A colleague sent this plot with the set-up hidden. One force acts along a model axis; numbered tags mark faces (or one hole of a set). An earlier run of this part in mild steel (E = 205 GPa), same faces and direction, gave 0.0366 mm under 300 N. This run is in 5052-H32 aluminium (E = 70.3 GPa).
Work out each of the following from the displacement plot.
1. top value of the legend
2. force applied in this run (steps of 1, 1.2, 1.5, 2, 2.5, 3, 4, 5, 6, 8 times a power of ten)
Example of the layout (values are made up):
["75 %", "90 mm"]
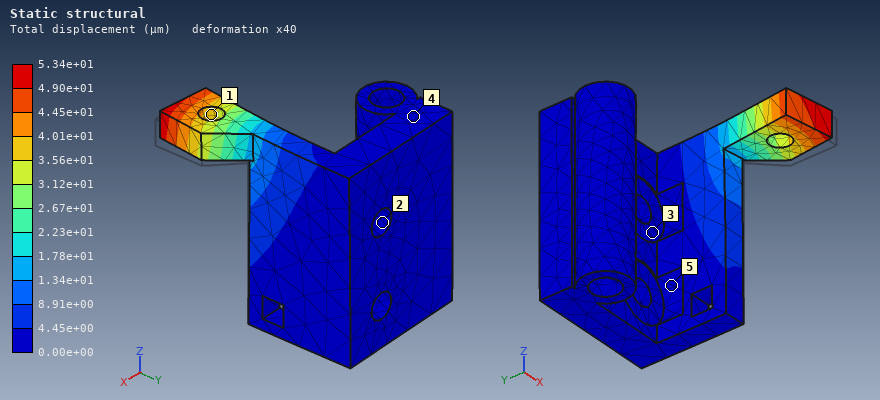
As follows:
["5.34e+01 µm", "150 N"]
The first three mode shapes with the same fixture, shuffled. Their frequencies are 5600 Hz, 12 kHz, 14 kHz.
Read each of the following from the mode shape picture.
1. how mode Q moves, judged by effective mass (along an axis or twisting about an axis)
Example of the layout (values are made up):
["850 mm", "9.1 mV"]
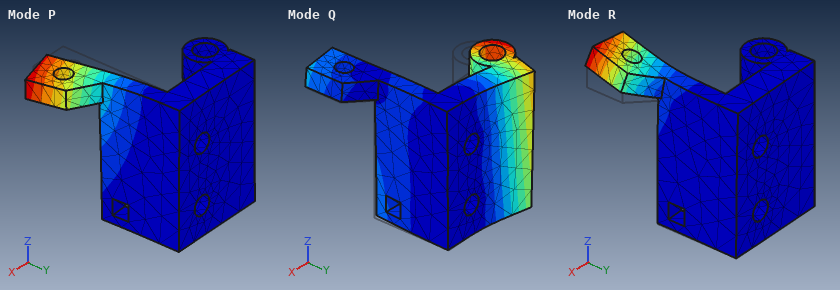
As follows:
["along Y"]
